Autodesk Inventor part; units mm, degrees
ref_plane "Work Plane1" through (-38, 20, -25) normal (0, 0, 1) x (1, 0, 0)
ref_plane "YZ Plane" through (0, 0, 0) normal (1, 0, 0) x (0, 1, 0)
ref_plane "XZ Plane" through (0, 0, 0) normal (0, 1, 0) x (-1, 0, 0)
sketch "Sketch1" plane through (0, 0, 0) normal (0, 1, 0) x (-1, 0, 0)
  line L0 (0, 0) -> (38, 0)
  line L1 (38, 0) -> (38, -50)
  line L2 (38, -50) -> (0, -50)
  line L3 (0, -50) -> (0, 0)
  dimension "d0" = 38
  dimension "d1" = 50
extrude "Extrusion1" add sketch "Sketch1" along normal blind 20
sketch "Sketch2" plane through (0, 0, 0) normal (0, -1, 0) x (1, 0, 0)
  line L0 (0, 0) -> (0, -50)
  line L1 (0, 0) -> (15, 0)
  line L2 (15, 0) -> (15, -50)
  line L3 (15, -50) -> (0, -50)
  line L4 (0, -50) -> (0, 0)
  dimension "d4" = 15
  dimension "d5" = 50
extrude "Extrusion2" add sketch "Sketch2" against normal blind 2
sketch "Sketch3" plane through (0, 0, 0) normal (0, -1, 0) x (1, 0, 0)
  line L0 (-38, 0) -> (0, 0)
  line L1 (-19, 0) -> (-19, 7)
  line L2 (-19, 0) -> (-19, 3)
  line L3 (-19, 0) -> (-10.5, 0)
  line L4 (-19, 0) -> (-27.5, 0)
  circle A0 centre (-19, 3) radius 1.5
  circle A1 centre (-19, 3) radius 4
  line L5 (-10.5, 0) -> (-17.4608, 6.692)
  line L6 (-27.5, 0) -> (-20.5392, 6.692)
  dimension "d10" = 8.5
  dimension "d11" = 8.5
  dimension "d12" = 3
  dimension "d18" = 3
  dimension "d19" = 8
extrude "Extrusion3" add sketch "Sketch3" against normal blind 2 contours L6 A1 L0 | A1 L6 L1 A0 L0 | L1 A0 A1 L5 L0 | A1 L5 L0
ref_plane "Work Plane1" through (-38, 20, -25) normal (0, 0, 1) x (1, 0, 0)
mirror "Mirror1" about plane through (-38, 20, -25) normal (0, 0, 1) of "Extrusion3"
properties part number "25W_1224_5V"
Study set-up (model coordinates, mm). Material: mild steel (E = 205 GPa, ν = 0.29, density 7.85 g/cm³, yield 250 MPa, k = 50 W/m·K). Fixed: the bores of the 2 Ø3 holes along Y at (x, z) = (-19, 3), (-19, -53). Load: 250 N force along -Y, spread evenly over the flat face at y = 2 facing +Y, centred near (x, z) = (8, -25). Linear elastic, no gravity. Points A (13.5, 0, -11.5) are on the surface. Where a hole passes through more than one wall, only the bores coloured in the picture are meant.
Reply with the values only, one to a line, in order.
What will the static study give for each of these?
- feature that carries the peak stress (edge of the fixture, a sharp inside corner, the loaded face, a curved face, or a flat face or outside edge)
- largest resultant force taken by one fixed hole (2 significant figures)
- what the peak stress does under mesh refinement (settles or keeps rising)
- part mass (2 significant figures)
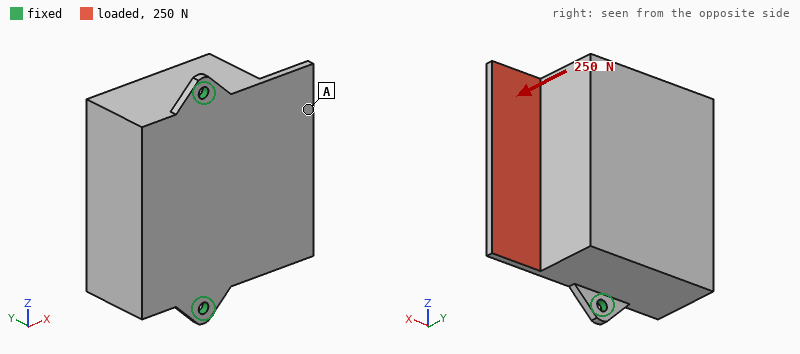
edge of the fixture
150 N
keeps rising
310 g
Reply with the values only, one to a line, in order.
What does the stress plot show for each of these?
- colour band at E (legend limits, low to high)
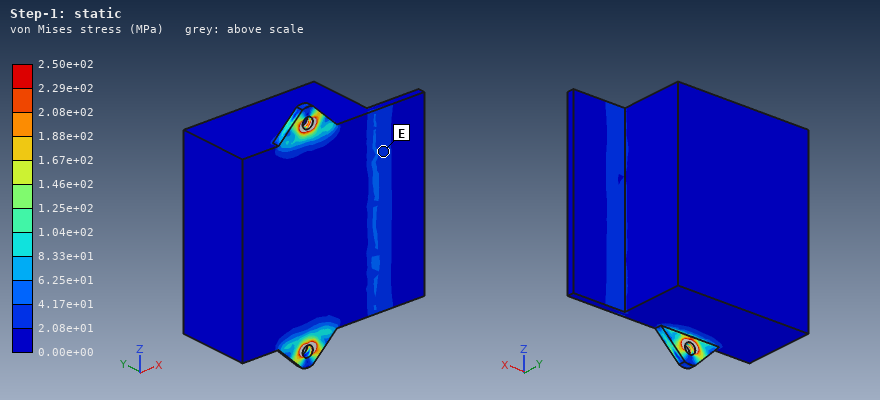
2.08e+01 to 4.17e+01 MPa
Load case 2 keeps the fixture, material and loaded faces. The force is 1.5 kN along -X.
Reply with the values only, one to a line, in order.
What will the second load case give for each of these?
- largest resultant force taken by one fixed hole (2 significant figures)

750 N
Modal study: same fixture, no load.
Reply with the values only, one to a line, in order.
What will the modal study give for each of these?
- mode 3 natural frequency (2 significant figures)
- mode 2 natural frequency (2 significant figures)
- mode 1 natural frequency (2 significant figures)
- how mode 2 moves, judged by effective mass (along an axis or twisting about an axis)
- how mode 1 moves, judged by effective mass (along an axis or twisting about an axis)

6900 Hz
5000 Hz
850 Hz
along Y
along X
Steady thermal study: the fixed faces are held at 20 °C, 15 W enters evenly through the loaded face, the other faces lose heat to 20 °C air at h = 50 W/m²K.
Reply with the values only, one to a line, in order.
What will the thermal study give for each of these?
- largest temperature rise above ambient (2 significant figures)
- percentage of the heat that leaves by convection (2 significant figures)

46 K
53 %
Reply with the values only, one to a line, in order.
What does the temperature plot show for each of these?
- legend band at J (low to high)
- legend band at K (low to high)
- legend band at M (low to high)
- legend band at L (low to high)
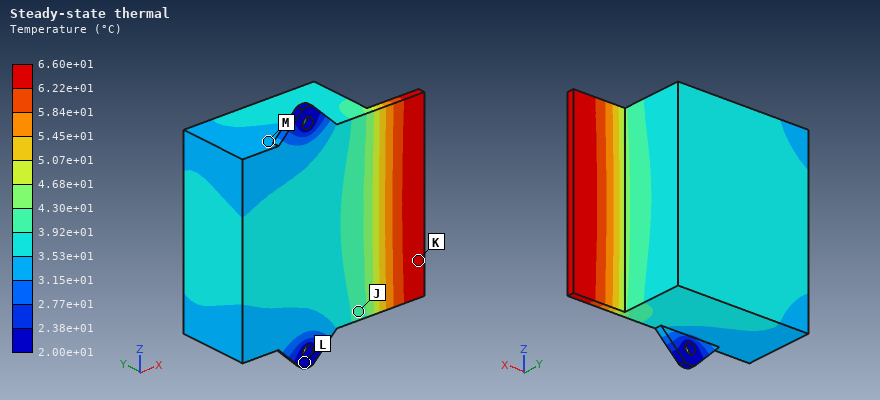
3.92e+01 to 4.30e+01 °C
6.22e+01 to 6.60e+01 °C
3.15e+01 to 3.53e+01 °C
2.00e+01 to 2.38e+01 °C
